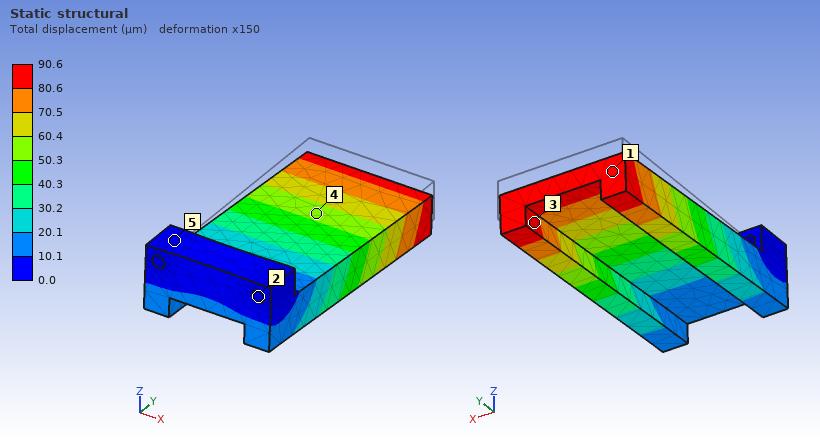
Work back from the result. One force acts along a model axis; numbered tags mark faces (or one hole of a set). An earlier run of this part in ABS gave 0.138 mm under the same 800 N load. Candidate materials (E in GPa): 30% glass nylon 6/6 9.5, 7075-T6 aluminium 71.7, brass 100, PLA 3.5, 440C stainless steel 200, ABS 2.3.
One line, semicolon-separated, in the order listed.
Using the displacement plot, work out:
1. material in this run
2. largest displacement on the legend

PLA; 90.6 µm
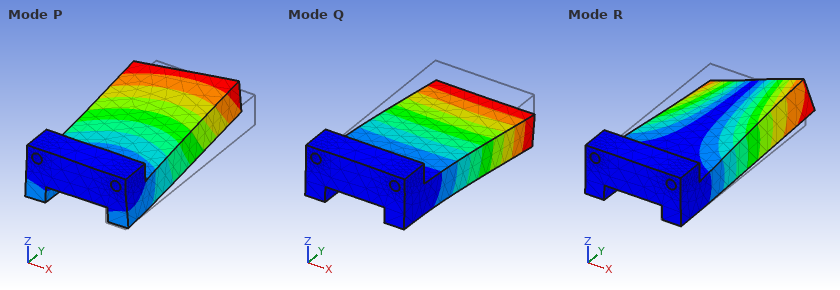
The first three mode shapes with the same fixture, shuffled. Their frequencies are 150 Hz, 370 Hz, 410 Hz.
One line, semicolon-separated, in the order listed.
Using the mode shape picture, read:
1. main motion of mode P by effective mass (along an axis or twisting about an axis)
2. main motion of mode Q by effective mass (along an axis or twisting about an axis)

along X; along Z
